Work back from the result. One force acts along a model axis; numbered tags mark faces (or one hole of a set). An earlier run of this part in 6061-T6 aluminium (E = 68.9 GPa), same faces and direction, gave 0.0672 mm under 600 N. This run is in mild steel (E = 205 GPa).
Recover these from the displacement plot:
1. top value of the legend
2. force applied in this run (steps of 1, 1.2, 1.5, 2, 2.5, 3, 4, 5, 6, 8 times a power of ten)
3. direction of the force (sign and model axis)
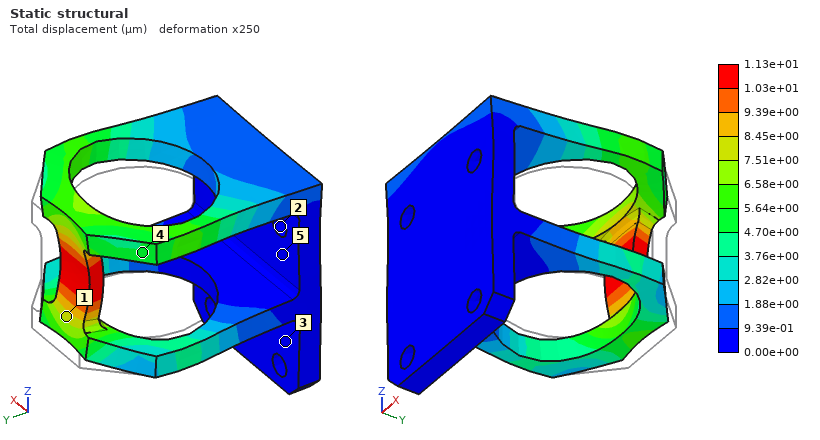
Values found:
1.13e+01 µm
300 N
-Y
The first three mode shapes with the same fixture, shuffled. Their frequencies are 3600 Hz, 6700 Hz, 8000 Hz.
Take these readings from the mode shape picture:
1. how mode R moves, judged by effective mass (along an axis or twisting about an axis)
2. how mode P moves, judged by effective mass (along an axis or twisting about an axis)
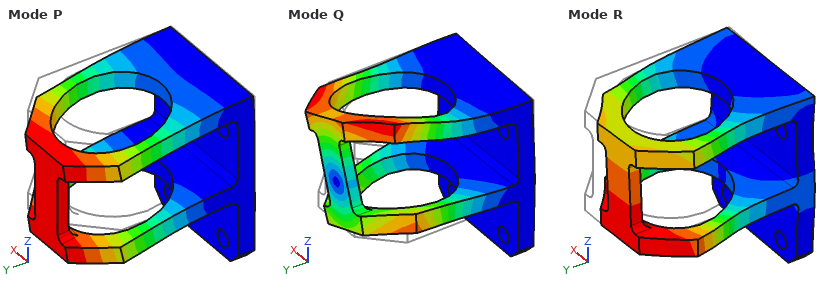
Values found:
along X
along Z
